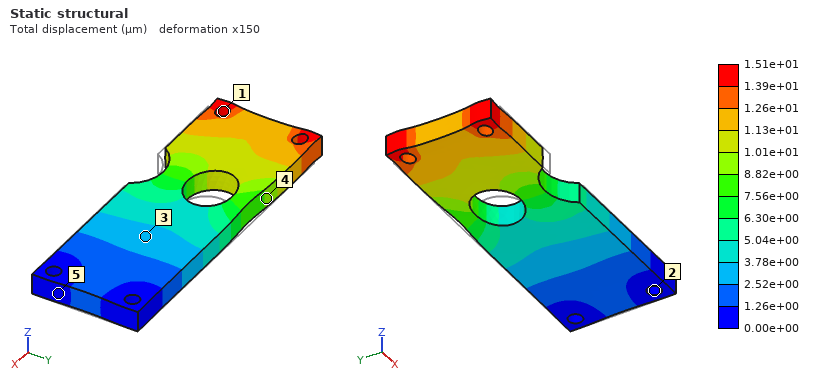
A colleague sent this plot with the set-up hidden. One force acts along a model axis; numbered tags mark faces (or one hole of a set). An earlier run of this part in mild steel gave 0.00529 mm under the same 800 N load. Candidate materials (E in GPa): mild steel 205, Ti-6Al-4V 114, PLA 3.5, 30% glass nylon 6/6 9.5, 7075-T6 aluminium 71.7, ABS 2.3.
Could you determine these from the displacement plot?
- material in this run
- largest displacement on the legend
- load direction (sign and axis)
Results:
7075-T6 aluminium
1.51e+01 µm
-X
